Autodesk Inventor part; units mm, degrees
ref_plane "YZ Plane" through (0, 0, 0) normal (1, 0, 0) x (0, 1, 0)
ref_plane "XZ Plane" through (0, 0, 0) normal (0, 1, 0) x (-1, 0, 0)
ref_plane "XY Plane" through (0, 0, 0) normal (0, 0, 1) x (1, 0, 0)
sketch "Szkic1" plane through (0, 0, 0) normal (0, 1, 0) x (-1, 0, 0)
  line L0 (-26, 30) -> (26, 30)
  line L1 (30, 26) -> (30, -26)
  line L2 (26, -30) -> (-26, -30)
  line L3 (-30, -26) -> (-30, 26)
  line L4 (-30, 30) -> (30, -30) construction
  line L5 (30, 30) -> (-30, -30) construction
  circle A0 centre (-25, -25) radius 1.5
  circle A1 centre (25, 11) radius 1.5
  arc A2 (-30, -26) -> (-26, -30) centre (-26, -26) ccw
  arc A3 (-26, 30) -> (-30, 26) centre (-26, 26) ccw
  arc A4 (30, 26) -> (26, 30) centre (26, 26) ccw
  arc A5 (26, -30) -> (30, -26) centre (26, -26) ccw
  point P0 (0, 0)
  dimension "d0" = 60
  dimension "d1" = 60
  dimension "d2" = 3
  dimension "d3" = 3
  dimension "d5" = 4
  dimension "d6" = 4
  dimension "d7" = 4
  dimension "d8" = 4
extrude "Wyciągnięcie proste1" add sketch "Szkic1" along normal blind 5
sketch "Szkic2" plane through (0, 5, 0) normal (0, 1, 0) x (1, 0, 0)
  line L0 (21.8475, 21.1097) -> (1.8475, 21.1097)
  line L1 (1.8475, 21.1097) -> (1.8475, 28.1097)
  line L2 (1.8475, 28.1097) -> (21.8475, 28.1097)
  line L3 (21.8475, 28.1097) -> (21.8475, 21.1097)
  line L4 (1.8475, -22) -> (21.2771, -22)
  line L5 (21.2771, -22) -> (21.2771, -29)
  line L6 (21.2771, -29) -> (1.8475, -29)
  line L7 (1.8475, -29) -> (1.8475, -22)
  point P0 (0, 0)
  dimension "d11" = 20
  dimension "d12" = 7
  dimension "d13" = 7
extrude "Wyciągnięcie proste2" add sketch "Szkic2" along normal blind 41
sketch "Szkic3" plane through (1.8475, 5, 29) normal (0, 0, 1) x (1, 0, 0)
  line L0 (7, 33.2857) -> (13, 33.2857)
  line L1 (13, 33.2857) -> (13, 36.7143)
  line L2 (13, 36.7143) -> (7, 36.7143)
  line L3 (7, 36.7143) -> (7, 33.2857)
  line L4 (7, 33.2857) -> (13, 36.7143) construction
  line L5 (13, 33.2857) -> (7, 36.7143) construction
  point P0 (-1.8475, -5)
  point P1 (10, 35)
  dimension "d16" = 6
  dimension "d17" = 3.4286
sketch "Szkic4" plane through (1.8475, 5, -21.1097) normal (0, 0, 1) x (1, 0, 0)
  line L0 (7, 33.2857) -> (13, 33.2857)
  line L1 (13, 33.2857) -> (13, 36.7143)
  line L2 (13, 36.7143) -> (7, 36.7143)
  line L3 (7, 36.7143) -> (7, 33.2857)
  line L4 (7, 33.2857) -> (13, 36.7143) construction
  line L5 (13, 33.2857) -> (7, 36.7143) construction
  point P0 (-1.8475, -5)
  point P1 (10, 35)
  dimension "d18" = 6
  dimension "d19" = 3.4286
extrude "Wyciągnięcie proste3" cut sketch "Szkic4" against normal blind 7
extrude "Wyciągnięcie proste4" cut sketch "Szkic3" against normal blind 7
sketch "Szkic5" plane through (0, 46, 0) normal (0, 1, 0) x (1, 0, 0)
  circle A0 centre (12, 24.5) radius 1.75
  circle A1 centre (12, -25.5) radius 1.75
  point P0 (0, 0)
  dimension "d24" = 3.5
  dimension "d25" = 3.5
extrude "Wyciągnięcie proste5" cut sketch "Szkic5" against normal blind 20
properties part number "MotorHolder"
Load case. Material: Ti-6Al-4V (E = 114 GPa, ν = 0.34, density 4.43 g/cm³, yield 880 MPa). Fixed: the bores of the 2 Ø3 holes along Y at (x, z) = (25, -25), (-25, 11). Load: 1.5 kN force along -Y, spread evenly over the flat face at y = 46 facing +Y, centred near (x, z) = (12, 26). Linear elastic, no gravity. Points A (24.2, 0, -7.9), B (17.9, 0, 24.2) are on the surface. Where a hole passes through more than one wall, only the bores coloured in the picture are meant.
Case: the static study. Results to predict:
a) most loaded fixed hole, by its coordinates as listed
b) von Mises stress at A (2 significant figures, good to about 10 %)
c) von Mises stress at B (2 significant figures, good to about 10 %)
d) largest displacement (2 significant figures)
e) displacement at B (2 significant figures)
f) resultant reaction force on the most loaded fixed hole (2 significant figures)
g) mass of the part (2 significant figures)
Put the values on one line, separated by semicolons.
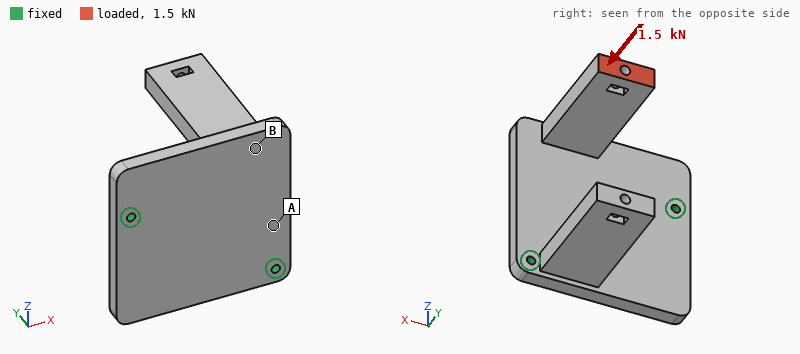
(-25, 11); 140 MPa; 69 MPa; 1.0 mm; 0.54 mm; 1.0 kN; 130 g
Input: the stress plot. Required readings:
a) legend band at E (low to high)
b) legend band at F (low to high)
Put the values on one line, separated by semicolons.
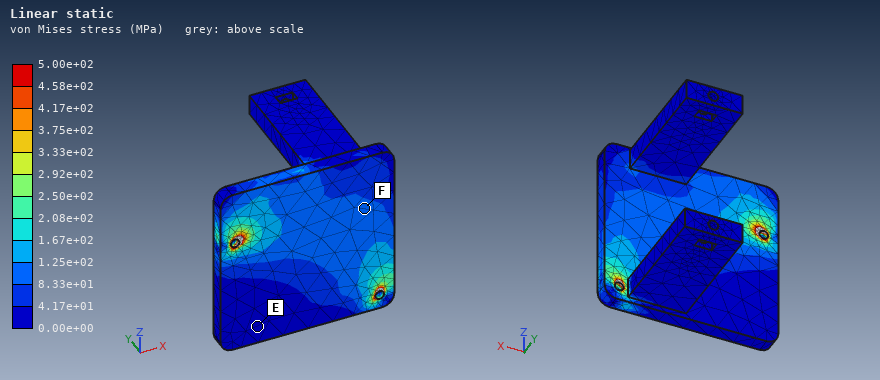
0.00e+00 to 4.17e+01 MPa; 8.33e+01 to 1.25e+02 MPa
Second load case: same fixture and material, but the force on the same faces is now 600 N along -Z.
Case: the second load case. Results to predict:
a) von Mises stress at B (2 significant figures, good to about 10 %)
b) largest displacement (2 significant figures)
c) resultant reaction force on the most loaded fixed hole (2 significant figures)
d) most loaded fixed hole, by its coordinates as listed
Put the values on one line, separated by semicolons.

94 MPa; 0.91 mm; 500 N; (25, -25)
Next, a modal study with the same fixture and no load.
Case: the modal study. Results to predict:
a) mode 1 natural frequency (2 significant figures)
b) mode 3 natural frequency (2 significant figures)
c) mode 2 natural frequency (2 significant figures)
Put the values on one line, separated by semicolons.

1100 Hz; 2300 Hz; 2000 Hz
